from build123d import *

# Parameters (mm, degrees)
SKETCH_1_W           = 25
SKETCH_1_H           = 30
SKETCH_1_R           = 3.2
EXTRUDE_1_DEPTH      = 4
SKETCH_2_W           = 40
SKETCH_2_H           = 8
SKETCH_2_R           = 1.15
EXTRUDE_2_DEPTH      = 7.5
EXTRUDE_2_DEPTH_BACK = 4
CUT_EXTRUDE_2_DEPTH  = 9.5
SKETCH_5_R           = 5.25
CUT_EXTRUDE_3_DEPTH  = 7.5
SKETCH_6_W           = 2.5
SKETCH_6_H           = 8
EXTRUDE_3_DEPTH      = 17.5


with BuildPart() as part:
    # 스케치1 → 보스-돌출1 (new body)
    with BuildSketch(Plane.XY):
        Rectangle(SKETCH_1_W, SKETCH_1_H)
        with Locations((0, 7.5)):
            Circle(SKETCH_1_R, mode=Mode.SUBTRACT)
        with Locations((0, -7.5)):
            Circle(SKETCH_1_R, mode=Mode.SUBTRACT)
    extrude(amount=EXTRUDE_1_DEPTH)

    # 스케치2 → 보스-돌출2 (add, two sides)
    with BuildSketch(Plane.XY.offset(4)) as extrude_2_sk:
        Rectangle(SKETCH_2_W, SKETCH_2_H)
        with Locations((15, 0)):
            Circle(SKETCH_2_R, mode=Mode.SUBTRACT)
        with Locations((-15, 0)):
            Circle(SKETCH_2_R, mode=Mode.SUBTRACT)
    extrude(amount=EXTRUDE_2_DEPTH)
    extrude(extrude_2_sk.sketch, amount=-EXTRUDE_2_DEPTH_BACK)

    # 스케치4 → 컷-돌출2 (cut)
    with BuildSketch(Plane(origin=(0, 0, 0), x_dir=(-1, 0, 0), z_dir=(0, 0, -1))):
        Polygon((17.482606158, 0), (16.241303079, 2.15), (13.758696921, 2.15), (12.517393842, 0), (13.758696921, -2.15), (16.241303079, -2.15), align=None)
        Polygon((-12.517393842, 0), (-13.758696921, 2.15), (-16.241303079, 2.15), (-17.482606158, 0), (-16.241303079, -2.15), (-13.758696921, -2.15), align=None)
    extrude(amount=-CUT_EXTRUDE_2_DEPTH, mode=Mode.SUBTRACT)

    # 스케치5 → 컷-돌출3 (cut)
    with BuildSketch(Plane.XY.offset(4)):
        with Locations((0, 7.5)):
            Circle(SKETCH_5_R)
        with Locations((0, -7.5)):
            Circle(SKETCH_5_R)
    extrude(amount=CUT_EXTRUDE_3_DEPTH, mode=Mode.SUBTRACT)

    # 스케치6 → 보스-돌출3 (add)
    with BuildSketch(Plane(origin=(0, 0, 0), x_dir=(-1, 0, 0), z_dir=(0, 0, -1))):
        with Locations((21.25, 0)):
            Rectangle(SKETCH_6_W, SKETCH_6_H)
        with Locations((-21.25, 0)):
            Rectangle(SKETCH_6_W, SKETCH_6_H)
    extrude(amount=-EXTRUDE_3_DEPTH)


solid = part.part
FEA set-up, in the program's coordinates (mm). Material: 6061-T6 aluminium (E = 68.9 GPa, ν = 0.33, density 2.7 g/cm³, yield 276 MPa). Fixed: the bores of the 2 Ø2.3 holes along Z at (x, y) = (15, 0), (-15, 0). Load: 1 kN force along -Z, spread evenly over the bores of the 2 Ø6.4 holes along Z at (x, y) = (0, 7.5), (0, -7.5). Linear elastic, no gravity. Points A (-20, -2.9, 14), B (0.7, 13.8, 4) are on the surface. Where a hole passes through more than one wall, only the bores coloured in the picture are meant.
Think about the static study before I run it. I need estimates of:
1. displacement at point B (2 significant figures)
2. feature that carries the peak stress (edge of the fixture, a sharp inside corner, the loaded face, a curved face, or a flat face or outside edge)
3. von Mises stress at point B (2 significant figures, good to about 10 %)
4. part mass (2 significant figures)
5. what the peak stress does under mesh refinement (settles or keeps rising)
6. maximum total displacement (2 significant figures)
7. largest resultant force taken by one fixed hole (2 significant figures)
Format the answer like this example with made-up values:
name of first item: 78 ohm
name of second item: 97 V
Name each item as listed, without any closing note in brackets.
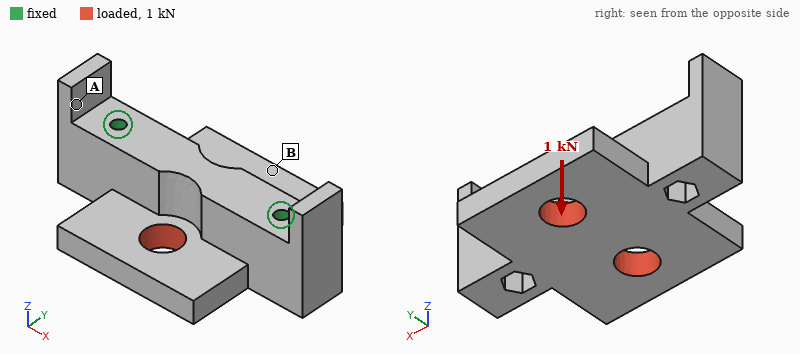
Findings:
displacement at point B: 22 µm
feature that carries the peak stress: edge of the fixture
von Mises stress at point B: 31 MPa
part mass: 16 g
what the peak stress does under mesh refinement: keeps rising
maximum total displacement: 24 µm
largest resultant force taken by one fixed hole: 660 N
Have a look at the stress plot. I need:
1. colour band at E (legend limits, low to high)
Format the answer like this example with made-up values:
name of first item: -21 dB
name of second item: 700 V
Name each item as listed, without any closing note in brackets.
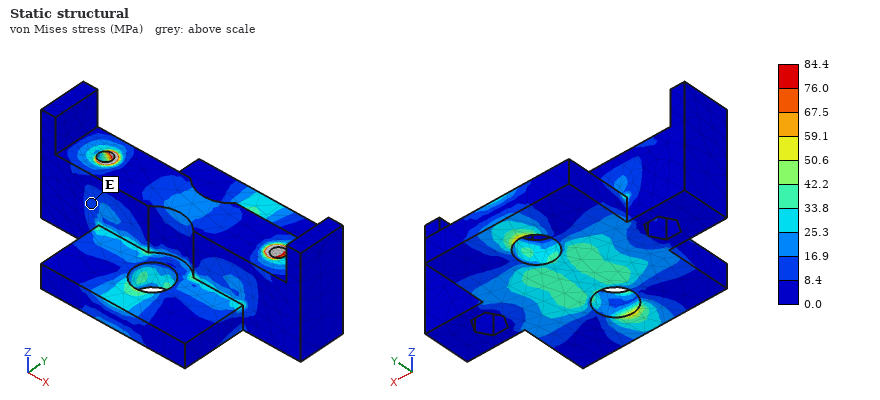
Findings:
colour band at E: 8.4 to 16.9 MPa
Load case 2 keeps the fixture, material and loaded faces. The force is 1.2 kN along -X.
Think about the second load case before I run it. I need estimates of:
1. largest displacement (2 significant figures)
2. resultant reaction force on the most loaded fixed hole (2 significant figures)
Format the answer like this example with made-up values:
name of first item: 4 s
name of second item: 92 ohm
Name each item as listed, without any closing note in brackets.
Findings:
largest displacement: 7.7 µm
resultant reaction force on the most loaded fixed hole: 690 N
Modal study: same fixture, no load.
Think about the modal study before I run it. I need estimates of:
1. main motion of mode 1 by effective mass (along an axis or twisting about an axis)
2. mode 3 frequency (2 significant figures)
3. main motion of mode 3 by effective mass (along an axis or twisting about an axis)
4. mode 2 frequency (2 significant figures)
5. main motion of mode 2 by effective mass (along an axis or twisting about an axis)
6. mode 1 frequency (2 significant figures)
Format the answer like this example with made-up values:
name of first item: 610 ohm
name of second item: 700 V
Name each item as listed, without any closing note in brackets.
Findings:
main motion of mode 1 by effective mass: along Y
mode 3 frequency: 15 kHz
main motion of mode 3 by effective mass: along Z
mode 2 frequency: 13 kHz
main motion of mode 2 by effective mass: twisting about Z
mode 1 frequency: 4500 Hz
